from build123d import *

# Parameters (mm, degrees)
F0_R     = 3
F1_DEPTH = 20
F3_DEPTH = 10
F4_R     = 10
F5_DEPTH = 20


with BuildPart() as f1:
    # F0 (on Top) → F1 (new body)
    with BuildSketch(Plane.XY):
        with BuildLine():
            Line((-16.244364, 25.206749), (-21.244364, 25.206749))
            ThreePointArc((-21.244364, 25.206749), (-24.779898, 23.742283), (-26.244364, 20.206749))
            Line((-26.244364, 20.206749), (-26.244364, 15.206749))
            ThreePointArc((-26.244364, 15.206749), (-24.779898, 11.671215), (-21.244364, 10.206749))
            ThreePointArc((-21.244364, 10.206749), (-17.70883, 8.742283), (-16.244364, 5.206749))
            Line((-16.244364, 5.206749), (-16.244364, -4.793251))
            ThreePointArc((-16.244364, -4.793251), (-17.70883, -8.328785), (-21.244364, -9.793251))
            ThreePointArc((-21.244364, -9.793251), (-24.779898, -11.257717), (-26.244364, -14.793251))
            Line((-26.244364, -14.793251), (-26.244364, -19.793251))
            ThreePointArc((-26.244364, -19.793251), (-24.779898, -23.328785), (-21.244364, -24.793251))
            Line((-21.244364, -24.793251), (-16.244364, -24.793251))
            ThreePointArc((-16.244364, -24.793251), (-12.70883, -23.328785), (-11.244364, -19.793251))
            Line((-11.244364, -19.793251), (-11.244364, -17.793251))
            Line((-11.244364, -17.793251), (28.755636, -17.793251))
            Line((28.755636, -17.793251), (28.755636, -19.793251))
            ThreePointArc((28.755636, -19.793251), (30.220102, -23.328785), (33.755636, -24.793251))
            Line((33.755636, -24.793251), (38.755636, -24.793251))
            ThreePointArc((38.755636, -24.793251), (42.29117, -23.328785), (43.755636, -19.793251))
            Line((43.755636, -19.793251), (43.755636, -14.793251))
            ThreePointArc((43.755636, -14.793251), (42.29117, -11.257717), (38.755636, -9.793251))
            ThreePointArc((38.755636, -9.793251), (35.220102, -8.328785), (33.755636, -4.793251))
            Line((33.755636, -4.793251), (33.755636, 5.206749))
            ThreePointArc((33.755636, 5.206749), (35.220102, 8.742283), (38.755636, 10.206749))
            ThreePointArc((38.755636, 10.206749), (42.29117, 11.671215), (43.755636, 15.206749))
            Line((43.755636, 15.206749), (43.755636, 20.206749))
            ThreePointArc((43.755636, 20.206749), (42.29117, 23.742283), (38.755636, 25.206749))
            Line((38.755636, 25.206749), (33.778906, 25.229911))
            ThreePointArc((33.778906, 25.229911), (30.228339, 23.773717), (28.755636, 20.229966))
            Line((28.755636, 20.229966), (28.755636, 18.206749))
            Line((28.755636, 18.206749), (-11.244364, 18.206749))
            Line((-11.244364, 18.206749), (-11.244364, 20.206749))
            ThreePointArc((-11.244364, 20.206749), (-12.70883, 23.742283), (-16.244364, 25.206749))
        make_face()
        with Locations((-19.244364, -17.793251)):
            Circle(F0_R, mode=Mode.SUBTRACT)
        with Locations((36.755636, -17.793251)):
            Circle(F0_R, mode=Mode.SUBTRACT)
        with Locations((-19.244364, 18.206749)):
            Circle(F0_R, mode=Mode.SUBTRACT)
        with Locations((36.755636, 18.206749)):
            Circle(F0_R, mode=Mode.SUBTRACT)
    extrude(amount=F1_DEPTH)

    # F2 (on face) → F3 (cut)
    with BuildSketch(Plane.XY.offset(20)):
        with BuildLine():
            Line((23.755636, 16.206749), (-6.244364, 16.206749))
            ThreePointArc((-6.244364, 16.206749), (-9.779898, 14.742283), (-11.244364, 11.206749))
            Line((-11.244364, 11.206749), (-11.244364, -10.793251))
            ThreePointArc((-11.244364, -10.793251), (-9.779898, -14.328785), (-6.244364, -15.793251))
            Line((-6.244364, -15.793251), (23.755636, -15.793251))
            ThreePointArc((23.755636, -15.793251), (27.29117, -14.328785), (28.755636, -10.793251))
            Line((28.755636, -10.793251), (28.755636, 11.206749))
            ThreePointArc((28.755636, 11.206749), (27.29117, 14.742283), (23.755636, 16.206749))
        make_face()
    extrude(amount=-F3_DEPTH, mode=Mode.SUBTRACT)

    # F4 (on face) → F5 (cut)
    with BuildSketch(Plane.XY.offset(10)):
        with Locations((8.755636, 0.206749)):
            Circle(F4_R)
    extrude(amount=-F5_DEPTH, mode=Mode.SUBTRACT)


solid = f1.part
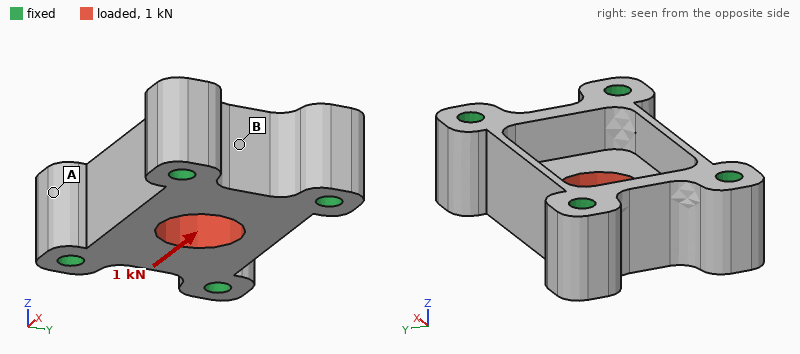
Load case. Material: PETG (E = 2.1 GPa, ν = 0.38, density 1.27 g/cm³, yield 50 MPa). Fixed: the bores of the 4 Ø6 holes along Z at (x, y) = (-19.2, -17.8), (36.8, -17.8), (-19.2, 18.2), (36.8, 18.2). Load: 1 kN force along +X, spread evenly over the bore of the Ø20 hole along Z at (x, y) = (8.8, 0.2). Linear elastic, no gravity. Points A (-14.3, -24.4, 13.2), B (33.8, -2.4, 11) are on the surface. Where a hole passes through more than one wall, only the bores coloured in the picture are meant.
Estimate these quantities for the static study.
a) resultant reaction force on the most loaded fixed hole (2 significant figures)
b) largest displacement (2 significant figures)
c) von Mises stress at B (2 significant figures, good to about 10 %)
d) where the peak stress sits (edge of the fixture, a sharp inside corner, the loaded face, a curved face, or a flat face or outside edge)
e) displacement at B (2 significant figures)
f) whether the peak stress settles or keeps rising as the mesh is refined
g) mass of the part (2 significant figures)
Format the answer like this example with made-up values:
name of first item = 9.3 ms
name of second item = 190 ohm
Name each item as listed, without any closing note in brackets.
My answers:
resultant reaction force on the most loaded fixed hole = 280 N
largest displacement = 23 µm
von Mises stress at B = 0.67 MPa
where the peak stress sits = edge of the fixture
displacement at B = 12 µm
whether the peak stress settles or keeps rising as the mesh is refined = keeps rising
mass of the part = 41 g
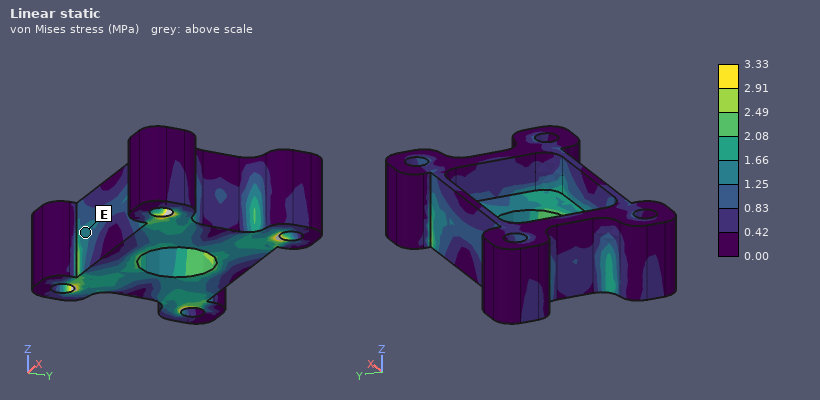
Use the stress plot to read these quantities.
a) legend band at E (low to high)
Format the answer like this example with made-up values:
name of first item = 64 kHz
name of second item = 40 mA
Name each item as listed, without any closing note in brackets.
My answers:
legend band at E = 1.25 to 1.66 MPa
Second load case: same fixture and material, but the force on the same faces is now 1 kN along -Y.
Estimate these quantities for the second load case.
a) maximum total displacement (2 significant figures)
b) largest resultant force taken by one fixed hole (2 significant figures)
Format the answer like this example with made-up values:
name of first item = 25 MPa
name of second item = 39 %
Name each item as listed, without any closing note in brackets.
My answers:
maximum total displacement = 60 µm
largest resultant force taken by one fixed hole = 320 N
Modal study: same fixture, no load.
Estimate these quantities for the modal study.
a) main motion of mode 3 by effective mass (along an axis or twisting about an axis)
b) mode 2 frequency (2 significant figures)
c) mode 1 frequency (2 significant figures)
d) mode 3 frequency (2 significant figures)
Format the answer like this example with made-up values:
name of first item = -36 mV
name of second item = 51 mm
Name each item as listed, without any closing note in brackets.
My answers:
main motion of mode 3 by effective mass = along Z
mode 2 frequency = 4500 Hz
mode 1 frequency = 4500 Hz
mode 3 frequency = 5200 Hz
